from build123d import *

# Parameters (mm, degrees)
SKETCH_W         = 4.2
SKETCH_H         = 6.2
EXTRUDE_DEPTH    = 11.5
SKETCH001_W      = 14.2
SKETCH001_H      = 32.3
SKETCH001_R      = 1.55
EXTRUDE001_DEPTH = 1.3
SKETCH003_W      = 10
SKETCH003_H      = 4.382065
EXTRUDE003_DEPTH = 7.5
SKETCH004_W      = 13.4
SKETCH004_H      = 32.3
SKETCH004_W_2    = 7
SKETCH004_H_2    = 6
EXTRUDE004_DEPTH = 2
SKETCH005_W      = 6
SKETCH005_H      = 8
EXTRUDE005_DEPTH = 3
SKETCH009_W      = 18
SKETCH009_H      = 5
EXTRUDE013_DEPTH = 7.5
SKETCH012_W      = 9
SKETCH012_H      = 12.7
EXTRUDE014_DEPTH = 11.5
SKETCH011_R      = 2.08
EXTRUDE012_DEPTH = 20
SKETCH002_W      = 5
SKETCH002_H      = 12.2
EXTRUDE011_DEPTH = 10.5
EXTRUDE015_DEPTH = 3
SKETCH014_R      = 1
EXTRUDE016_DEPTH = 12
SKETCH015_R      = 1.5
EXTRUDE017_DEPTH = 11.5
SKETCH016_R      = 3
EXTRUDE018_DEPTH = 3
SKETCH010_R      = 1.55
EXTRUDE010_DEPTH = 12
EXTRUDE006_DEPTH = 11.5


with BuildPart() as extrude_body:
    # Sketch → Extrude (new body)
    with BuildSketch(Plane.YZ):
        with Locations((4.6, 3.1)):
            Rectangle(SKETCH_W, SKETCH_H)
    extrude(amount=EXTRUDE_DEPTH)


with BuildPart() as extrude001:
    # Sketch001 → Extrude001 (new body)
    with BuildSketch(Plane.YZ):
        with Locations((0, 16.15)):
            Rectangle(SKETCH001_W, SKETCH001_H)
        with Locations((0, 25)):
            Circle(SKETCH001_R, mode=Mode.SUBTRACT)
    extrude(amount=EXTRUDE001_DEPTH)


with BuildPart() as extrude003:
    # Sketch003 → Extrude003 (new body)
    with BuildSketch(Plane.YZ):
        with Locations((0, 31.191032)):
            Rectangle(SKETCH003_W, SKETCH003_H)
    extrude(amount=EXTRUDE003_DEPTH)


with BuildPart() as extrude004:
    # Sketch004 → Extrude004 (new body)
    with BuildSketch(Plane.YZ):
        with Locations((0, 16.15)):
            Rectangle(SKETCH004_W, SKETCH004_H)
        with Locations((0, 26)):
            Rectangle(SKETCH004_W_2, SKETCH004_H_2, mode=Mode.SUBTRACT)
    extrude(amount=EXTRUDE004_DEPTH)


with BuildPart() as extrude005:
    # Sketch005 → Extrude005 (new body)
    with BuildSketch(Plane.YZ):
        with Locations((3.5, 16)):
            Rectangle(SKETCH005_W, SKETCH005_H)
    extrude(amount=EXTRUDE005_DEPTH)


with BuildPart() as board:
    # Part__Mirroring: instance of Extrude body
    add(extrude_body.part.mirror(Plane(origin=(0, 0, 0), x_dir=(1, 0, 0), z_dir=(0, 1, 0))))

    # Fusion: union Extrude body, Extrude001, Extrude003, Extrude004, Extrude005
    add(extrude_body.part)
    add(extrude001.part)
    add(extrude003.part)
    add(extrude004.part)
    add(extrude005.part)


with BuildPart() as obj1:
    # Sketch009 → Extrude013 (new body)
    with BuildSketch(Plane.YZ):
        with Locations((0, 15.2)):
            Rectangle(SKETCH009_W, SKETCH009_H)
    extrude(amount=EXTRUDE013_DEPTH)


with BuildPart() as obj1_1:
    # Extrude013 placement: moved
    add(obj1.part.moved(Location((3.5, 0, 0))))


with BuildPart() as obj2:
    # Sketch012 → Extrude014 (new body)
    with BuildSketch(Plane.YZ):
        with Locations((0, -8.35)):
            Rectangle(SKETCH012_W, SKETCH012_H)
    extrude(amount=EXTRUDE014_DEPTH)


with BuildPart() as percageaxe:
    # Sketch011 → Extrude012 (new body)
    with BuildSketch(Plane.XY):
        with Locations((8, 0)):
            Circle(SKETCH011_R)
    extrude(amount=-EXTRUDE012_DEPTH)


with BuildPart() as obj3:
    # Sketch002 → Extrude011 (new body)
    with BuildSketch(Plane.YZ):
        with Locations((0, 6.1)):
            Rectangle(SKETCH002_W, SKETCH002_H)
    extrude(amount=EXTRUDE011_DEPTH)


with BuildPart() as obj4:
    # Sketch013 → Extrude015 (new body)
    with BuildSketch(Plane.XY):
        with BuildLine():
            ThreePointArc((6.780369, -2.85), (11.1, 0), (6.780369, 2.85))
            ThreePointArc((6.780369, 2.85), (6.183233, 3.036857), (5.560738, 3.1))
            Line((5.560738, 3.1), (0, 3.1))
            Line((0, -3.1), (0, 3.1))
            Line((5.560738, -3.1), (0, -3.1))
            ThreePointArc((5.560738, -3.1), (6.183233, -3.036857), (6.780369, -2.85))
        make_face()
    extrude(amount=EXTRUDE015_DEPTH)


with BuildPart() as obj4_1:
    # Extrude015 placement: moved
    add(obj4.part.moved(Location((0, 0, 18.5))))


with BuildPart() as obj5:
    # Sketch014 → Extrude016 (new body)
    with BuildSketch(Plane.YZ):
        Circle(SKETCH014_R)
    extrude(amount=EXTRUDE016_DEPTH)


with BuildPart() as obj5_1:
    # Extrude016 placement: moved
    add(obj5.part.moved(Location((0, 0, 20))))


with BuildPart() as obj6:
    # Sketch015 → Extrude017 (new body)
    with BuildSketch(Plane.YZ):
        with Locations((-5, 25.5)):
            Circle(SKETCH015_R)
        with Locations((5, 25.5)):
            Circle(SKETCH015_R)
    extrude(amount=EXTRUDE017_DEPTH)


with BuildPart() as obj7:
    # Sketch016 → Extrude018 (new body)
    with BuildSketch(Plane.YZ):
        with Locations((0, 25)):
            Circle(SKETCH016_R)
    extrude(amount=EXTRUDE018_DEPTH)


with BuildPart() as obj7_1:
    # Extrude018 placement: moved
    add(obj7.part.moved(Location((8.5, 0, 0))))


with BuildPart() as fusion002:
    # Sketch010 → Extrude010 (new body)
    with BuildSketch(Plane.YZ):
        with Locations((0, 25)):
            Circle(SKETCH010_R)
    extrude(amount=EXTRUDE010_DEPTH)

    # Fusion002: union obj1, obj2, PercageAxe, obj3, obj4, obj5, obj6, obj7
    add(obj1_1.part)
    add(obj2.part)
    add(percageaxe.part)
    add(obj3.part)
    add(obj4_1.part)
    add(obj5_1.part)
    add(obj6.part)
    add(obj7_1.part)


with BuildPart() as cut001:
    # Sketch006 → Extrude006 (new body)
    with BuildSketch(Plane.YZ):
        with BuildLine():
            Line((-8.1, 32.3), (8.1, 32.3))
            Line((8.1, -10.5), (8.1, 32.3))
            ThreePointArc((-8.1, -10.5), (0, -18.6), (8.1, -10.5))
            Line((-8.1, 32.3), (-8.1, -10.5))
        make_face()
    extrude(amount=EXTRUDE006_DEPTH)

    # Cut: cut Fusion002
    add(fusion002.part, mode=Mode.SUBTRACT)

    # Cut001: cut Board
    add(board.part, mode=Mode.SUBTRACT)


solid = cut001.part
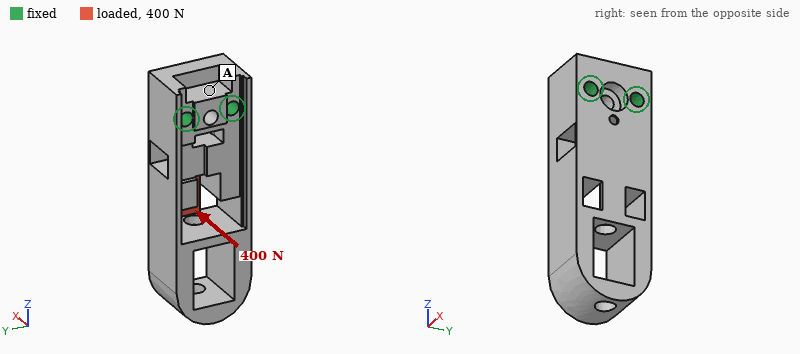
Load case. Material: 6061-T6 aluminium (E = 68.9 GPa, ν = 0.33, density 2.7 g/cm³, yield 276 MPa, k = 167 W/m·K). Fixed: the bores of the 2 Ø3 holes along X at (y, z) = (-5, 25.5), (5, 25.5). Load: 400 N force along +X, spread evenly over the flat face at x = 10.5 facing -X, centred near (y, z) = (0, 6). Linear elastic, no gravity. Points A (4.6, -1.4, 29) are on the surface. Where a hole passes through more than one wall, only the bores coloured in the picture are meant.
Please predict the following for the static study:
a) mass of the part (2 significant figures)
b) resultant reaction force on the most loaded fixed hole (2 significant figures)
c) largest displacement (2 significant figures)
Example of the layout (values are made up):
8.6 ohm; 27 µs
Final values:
12 g; 210 N; 93 µm
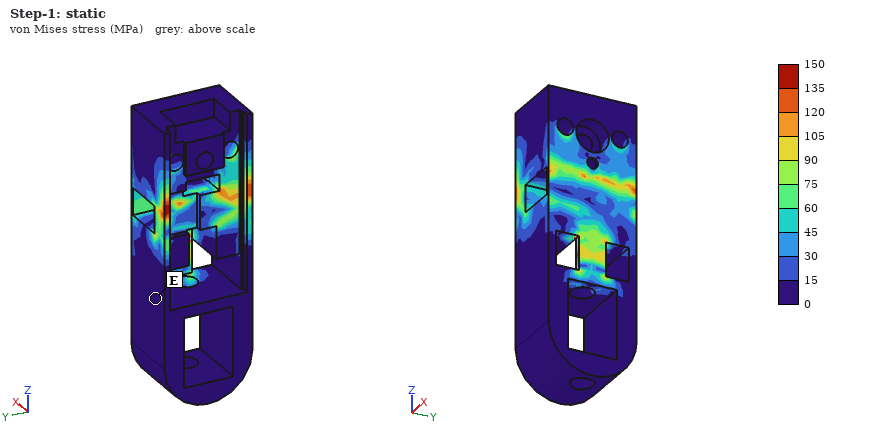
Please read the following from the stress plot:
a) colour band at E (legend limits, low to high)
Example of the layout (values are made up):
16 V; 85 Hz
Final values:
0 to 15 MPa
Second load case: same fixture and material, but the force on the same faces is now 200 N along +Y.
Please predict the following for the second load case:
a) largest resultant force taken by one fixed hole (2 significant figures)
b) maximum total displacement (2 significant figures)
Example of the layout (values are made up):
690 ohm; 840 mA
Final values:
290 N; 29 µm
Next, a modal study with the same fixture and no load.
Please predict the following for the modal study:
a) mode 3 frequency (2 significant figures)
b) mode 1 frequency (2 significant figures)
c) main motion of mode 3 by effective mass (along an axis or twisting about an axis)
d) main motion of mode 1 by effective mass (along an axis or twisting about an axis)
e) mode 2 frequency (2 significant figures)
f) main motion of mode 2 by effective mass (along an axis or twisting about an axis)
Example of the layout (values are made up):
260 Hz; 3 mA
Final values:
8100 Hz; 3400 Hz; twisting about Z; along X; 3800 Hz; along Y
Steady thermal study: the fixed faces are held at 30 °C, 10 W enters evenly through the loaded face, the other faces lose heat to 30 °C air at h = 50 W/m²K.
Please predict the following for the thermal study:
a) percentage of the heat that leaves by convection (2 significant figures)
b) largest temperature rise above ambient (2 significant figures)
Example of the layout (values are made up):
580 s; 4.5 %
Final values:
24 %; 29 K
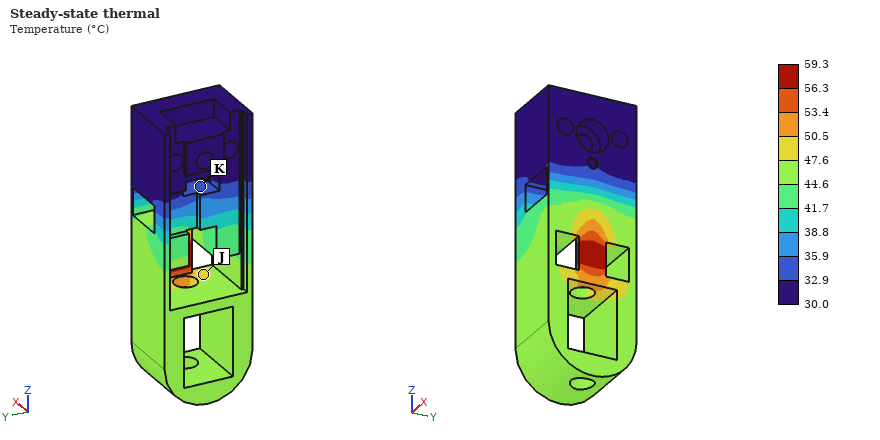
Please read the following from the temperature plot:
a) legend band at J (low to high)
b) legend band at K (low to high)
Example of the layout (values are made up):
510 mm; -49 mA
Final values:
47.6 to 50.5 °C; 32.9 to 35.9 °C
